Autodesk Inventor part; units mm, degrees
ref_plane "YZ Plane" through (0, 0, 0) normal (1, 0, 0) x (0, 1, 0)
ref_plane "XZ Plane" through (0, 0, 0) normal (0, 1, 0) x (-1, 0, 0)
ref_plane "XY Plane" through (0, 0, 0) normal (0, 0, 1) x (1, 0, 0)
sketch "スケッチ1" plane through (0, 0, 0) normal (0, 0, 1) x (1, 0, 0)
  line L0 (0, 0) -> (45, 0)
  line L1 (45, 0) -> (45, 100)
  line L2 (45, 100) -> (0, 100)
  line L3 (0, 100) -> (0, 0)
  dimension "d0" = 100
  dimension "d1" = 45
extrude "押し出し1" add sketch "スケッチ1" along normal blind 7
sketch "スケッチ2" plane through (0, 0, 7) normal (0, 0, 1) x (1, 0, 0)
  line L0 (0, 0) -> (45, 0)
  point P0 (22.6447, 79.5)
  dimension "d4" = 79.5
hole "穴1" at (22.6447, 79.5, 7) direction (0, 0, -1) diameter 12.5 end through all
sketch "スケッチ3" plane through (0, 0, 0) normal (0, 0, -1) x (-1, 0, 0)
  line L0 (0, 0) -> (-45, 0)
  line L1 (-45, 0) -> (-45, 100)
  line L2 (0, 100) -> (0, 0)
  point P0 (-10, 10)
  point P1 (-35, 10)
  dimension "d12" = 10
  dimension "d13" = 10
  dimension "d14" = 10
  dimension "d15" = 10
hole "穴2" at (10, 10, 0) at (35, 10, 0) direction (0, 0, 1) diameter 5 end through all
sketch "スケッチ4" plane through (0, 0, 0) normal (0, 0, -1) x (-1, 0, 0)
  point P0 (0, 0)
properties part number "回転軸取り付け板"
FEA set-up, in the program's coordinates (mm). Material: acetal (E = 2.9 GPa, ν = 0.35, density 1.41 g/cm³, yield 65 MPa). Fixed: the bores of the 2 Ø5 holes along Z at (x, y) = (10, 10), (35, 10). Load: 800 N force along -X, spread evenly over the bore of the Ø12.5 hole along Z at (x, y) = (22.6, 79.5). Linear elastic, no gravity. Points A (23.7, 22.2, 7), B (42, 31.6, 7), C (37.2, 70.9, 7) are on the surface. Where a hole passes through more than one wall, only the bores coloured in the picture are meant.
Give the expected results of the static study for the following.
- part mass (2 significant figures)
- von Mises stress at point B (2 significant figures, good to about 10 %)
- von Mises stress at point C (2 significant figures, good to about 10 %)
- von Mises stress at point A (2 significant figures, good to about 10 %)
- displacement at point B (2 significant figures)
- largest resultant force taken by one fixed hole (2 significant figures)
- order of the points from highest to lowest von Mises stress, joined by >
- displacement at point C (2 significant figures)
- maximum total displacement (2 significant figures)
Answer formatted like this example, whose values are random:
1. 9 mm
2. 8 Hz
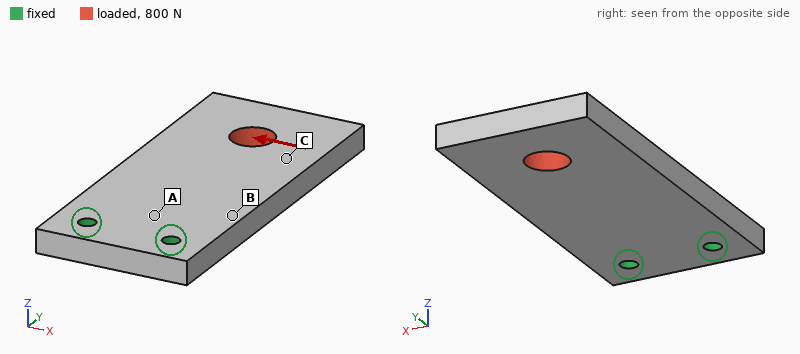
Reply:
1. 43 g
2. 14 MPa
3. 4.5 MPa
4. 8.9 MPa
5. 0.25 mm
6. 2.0 kN
7. B > A > C
8. 0.79 mm
9. 1.3 mm
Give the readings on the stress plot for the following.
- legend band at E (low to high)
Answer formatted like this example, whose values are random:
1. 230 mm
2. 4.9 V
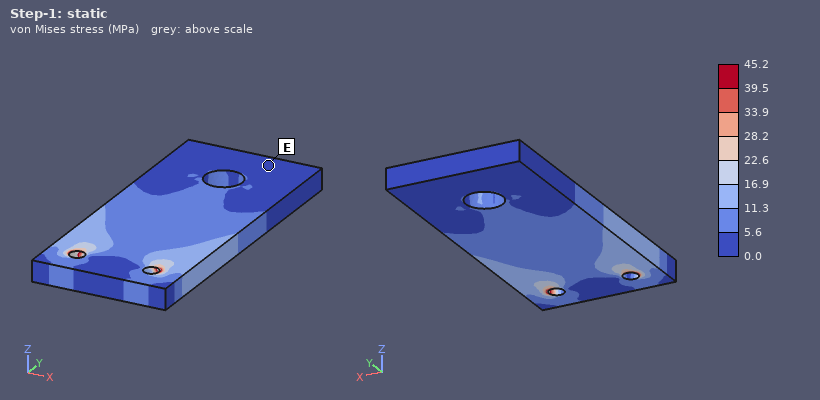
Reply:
1. 0.0 to 5.6 MPa
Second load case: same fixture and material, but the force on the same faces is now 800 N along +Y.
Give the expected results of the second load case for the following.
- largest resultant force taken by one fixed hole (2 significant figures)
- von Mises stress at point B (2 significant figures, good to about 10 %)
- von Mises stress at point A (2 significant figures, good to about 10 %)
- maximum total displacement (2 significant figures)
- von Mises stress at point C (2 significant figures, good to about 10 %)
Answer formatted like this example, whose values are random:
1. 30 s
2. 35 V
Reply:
1. 410 N
2. 2.5 MPa
3. 2.1 MPa
4. 87 µm
5. 2.5 MPa
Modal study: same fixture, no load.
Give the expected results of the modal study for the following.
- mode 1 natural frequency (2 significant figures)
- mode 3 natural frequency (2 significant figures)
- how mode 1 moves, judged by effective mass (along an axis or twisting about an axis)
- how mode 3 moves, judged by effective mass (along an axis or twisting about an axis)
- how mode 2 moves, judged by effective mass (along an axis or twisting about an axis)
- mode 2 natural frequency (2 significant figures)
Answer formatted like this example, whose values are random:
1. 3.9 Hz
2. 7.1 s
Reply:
1. 210 Hz
2. 1000 Hz
3. along Z
4. along X
5. twisting about Y
6. 790 Hz
